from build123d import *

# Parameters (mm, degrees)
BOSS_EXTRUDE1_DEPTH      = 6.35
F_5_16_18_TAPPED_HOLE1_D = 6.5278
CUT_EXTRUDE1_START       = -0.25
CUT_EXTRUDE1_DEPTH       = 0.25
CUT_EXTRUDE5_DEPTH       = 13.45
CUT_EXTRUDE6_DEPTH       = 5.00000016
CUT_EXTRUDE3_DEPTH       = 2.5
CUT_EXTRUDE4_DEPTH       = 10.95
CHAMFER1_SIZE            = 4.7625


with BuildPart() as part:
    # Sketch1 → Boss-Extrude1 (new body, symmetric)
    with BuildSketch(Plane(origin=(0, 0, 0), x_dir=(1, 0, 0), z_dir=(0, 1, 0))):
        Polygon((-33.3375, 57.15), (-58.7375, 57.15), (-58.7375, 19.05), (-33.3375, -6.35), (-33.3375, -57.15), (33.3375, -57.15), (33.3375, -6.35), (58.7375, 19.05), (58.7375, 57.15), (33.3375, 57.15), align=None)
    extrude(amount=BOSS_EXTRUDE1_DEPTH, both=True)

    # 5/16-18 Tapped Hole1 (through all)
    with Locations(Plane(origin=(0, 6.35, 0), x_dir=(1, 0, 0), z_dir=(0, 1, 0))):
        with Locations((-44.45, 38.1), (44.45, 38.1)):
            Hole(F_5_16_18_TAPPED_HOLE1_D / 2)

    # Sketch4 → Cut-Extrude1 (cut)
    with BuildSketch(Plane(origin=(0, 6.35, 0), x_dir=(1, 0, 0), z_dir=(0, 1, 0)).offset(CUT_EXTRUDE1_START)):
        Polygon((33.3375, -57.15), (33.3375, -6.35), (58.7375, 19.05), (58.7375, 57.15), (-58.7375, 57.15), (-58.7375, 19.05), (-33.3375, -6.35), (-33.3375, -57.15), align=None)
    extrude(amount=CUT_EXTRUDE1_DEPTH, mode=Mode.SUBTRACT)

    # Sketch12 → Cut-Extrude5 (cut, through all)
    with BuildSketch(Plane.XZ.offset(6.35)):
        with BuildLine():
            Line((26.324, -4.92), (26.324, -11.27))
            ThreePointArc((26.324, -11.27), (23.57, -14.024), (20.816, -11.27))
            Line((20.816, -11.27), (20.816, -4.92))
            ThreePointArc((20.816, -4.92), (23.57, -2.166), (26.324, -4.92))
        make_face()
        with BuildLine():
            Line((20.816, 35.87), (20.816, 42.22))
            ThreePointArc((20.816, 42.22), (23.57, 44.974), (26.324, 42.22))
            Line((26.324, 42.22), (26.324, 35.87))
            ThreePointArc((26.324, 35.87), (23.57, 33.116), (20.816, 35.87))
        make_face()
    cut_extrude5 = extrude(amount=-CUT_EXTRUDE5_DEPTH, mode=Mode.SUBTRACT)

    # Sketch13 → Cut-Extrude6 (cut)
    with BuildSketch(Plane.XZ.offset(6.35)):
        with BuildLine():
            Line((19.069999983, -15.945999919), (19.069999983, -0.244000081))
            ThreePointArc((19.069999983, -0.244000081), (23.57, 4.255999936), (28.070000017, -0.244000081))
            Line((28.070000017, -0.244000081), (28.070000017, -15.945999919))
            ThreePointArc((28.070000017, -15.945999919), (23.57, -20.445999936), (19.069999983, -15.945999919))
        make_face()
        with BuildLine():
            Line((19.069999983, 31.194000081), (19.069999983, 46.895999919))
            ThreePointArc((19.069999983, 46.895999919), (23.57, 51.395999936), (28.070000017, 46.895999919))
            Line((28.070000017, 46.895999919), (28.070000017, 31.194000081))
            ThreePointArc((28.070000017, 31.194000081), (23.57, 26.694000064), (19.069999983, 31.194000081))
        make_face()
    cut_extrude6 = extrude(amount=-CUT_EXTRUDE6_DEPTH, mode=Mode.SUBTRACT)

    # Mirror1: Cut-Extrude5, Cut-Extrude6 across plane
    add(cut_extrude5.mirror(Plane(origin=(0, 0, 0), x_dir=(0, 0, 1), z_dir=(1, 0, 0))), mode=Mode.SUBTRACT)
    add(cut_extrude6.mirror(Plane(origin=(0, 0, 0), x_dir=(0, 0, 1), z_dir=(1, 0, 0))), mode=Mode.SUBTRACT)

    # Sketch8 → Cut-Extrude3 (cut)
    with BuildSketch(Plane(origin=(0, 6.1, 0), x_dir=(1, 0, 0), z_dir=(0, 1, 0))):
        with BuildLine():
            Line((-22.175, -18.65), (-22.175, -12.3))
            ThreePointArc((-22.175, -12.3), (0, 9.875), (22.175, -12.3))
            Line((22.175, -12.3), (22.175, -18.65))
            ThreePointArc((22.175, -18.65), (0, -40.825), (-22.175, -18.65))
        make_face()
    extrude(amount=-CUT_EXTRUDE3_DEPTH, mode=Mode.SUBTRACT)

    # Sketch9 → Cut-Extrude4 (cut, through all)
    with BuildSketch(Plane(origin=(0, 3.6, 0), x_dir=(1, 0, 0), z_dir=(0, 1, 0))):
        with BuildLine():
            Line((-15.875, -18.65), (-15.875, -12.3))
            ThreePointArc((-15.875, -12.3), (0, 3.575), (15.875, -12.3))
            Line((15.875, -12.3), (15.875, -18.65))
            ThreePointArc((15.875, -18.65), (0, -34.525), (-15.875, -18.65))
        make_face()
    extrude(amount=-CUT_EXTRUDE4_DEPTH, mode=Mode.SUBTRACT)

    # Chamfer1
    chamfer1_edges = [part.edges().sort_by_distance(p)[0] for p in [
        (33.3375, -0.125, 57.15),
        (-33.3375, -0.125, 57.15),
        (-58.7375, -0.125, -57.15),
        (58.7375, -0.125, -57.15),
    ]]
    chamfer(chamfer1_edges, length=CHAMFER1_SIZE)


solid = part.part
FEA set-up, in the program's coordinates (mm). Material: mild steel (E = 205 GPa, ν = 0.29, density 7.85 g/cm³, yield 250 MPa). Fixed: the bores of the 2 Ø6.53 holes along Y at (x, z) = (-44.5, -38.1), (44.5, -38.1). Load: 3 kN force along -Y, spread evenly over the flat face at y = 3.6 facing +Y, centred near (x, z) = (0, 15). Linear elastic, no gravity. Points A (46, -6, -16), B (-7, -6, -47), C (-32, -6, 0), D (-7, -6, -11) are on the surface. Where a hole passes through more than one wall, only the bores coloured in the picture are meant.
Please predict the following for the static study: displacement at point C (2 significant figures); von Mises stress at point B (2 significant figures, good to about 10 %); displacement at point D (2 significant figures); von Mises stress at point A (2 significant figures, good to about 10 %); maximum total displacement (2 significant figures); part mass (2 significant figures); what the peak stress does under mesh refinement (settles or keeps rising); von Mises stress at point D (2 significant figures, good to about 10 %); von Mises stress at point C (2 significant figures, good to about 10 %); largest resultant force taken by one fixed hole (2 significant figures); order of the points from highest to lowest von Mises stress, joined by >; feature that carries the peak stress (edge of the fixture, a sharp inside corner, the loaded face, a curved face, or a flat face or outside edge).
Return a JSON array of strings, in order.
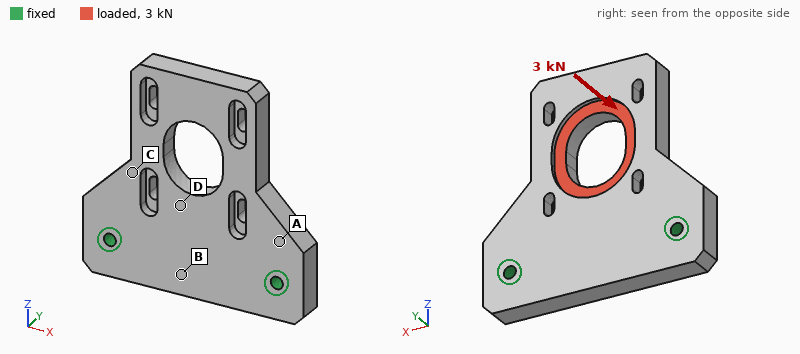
["0.050 mm", "12 MPa", "0.042 mm", "51 MPa", "0.21 mm", "830 g", "keeps rising", "31 MPa", "64 MPa", "1.5 kN", "C > A > D > B", "edge of the fixture"]
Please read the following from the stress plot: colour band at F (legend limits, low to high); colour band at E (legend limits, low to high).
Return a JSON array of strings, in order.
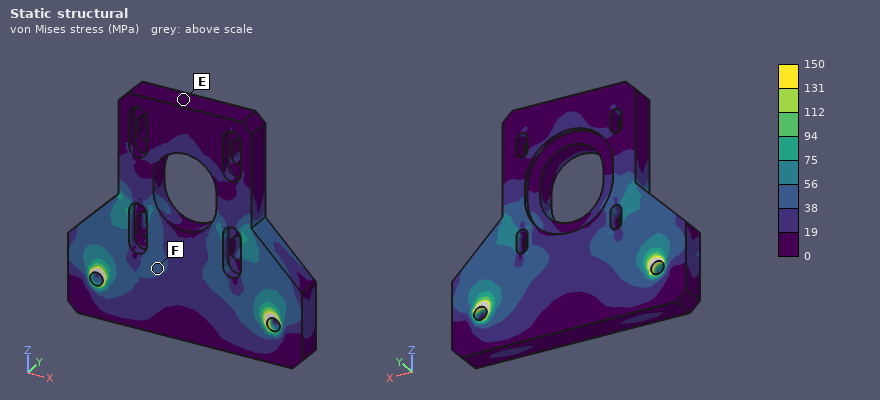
["38 to 56 MPa", "0 to 19 MPa"]
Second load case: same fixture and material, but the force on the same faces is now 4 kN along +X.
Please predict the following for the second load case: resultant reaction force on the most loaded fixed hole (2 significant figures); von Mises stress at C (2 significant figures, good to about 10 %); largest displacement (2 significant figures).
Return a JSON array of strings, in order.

["3.1 kN", "15 MPa", "17 µm"]
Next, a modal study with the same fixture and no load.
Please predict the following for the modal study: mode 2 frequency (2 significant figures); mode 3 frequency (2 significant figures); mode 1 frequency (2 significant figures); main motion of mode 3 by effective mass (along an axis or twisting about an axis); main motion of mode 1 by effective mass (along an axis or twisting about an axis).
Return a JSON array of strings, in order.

["3100 Hz", "4900 Hz", "1100 Hz", "along Y", "along Y"]
